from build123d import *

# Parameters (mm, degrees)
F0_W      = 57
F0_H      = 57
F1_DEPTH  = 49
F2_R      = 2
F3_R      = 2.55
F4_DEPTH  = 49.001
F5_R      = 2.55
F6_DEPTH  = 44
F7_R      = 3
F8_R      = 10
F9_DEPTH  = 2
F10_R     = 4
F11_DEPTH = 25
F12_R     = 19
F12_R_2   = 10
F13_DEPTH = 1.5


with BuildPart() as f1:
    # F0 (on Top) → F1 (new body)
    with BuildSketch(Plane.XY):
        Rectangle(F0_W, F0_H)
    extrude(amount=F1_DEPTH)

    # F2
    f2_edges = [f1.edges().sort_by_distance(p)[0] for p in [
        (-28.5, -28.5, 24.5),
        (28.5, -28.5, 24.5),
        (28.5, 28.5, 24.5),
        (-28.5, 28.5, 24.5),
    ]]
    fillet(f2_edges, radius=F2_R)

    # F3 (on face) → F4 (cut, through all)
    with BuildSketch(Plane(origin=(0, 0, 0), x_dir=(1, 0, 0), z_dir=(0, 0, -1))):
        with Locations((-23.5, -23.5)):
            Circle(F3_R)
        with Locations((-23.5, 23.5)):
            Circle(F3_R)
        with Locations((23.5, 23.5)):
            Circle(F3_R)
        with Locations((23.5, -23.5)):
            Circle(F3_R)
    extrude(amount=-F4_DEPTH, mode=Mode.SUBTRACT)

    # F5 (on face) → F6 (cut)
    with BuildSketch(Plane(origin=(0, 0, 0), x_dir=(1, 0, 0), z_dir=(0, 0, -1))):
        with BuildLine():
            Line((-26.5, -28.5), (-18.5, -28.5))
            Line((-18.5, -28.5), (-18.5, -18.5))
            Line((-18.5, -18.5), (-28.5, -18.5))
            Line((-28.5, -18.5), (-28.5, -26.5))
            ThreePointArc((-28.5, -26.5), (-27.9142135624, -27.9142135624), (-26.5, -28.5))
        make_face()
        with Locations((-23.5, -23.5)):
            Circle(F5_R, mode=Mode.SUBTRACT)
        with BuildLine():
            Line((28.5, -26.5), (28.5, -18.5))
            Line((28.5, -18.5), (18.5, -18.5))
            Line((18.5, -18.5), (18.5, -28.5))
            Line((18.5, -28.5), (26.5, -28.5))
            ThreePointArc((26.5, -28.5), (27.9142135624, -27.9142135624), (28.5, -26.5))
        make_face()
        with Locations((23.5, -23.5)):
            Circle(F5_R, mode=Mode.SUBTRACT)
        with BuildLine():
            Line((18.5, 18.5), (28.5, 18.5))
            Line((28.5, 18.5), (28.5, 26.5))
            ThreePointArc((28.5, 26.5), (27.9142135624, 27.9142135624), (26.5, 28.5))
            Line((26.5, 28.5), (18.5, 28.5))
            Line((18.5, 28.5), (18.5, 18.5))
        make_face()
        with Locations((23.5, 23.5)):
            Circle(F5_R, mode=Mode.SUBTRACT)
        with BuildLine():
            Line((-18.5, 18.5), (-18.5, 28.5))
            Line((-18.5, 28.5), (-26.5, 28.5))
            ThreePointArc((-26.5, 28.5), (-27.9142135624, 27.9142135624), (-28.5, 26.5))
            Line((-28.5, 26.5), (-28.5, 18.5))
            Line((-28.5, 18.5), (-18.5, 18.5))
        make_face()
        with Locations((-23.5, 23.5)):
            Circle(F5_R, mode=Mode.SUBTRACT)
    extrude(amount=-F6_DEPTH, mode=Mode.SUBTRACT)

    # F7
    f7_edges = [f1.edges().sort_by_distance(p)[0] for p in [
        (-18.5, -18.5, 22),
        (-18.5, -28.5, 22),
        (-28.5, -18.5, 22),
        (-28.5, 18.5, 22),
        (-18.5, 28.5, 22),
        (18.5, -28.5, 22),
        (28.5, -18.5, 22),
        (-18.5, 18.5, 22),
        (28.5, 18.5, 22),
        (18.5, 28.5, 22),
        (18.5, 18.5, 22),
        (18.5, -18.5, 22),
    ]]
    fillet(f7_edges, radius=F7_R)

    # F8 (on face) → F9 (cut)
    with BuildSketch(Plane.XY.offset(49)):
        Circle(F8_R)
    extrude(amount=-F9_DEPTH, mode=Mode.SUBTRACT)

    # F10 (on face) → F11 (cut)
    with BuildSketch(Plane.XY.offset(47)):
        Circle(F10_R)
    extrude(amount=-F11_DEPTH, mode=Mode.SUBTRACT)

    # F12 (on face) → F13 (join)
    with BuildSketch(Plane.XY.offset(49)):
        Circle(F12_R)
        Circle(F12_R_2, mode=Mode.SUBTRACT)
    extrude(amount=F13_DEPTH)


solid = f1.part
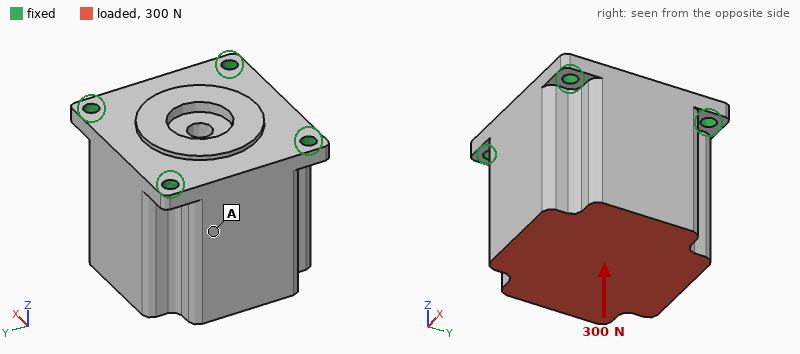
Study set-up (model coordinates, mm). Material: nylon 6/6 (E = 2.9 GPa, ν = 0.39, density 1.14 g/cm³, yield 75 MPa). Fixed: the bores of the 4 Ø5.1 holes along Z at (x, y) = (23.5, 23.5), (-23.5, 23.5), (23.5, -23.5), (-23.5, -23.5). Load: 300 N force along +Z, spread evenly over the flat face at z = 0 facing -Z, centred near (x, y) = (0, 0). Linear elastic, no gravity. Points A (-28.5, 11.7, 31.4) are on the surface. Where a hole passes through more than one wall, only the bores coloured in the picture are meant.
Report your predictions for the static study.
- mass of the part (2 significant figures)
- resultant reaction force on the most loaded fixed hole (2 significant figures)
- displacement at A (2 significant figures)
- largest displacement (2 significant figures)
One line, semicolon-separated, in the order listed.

160 g; 81 N; 7.9 µm; 9.3 µm
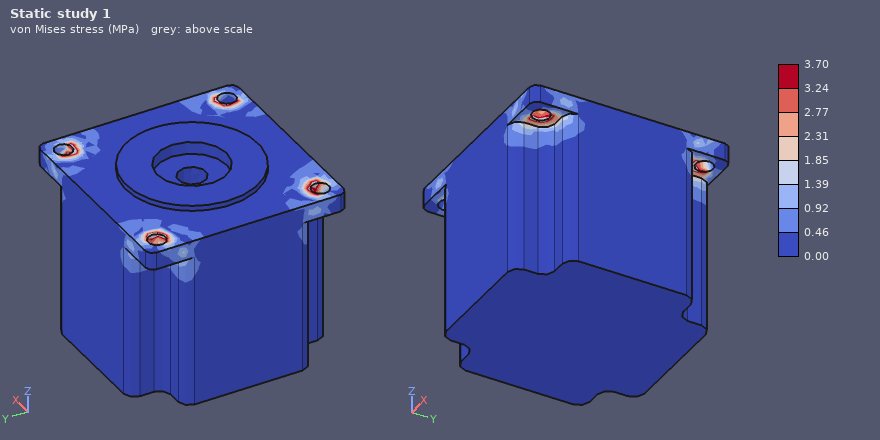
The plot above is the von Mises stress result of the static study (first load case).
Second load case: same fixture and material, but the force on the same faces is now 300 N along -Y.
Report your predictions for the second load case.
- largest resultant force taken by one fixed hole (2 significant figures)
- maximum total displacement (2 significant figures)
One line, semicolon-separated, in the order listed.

180 N; 51 µm
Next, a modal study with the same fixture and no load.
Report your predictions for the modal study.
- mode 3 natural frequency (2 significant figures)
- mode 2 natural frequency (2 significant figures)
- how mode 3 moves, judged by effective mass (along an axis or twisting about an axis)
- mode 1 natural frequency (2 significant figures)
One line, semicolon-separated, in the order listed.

2400 Hz; 1600 Hz; along Z; 1600 Hz
